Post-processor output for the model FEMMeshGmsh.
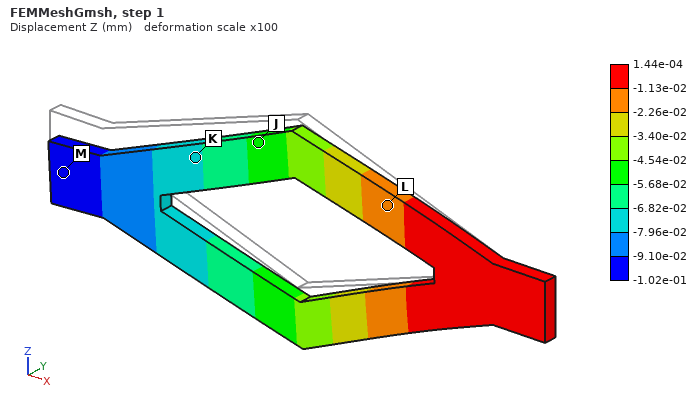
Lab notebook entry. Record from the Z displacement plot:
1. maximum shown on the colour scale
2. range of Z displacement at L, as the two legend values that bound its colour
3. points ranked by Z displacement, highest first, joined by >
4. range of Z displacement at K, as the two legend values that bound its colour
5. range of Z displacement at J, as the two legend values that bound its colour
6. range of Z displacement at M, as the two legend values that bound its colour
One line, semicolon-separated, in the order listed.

1.44e-04 mm; -2.26e-02 to -1.13e-02 mm; L > J > K > M; -7.96e-02 to -6.82e-02 mm; -5.68e-02 to -4.54e-02 mm; -1.02e-01 to -9.10e-02 mm
